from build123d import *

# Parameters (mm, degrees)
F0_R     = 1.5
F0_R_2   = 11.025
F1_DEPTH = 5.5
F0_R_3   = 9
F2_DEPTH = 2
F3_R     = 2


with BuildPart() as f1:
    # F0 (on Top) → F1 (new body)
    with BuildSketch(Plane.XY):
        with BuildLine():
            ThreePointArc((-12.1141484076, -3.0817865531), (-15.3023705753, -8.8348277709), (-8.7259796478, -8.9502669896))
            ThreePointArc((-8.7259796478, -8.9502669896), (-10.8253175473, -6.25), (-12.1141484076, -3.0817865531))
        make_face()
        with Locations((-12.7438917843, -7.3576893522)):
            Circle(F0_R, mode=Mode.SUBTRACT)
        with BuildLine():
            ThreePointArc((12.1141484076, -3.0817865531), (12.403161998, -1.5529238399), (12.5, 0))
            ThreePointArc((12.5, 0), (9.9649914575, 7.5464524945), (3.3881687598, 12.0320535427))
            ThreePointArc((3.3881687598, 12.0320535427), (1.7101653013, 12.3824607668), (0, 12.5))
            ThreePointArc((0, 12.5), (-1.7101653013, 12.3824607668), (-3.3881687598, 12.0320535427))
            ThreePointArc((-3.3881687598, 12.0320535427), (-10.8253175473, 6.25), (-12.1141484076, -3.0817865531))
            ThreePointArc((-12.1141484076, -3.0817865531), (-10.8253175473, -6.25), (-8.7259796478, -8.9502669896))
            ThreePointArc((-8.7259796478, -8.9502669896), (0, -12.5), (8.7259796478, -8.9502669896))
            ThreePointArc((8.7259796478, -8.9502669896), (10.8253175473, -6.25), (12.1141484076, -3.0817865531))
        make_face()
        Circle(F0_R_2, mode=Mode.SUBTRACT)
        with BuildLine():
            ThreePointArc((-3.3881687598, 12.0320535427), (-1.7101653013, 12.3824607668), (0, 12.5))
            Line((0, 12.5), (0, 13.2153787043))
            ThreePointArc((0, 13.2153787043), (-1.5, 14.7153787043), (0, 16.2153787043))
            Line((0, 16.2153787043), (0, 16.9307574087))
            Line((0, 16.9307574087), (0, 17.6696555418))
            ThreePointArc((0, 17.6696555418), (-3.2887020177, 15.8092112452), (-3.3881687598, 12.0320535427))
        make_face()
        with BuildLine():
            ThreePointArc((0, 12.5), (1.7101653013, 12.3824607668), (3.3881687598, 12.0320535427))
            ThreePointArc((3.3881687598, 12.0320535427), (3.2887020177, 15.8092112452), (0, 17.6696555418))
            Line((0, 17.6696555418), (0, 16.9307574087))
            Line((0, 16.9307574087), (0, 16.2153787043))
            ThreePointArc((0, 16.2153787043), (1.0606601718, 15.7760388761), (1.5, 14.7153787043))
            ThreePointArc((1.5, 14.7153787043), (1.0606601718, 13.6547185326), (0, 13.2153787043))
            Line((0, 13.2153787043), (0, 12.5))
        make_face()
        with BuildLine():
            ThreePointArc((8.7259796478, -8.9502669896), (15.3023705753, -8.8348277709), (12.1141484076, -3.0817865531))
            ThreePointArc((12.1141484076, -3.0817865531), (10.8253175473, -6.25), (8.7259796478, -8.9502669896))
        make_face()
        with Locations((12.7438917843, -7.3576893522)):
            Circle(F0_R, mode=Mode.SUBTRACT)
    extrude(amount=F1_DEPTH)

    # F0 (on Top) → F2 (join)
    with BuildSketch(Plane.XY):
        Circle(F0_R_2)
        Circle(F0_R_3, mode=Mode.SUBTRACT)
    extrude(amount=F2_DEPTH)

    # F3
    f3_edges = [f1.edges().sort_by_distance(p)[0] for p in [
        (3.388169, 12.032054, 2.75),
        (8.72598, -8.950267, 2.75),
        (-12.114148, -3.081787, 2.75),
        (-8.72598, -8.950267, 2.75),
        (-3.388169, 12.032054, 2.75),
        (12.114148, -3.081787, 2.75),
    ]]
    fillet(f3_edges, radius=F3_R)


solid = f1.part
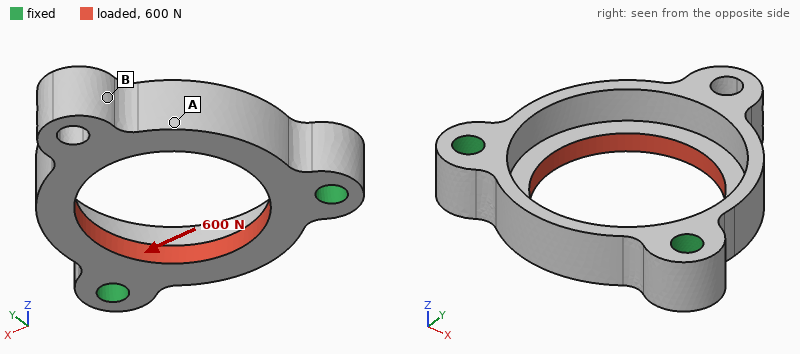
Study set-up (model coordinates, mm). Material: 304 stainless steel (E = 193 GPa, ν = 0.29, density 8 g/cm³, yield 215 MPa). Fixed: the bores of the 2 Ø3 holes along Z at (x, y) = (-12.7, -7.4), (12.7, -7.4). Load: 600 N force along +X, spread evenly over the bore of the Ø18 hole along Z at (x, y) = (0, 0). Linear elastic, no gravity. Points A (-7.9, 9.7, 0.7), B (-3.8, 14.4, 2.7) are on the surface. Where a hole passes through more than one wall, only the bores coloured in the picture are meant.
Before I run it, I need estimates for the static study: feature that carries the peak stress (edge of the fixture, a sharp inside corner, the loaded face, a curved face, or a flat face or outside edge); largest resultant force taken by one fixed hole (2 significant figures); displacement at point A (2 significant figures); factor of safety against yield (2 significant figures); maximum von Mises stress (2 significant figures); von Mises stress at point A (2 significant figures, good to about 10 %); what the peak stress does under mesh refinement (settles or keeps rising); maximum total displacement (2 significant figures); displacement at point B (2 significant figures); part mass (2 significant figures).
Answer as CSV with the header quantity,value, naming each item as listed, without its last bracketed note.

quantity,value
feature that carries the peak stress,a curved face
largest resultant force taken by one fixed hole,310 N
displacement at point A,15 µm
factor of safety against yield,1.5
maximum von Mises stress,150 MPa
von Mises stress at point A,60 MPa
what the peak stress does under mesh refinement,settles
maximum total displacement,16 µm
displacement at point B,12 µm
part mass,11 g
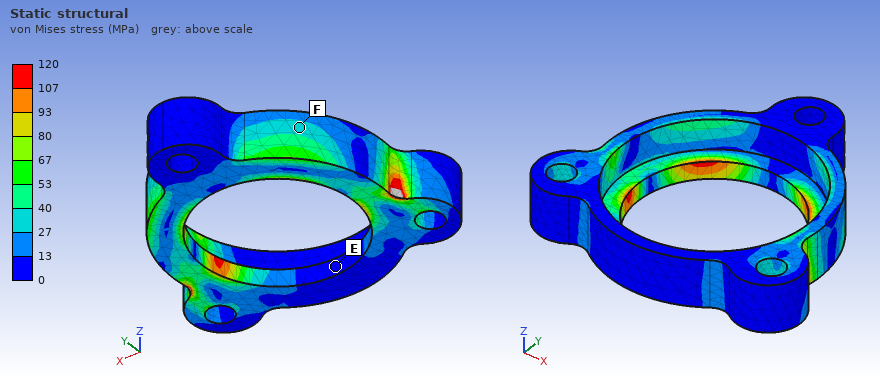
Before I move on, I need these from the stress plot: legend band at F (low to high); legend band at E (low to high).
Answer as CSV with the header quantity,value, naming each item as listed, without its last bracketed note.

quantity,value
legend band at F,27 to 40 MPa
legend band at E,0 to 13 MPa
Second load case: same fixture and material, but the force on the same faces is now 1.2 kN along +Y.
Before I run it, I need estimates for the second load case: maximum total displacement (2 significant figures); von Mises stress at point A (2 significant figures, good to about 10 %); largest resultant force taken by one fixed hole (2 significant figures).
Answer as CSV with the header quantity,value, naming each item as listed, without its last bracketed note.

quantity,value
maximum total displacement,18 µm
von Mises stress at point A,23 MPa
largest resultant force taken by one fixed hole,600 N
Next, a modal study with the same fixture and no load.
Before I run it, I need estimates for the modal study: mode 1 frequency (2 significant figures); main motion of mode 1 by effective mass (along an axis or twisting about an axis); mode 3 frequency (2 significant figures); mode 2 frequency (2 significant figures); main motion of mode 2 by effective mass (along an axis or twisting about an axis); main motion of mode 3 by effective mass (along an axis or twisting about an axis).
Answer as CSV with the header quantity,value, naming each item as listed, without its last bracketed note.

quantity,value
mode 1 frequency,5700 Hz
main motion of mode 1 by effective mass,along Z
mode 3 frequency,22 kHz
mode 2 frequency,11 kHz
main motion of mode 2 by effective mass,along X
main motion of mode 3 by effective mass,along Y
